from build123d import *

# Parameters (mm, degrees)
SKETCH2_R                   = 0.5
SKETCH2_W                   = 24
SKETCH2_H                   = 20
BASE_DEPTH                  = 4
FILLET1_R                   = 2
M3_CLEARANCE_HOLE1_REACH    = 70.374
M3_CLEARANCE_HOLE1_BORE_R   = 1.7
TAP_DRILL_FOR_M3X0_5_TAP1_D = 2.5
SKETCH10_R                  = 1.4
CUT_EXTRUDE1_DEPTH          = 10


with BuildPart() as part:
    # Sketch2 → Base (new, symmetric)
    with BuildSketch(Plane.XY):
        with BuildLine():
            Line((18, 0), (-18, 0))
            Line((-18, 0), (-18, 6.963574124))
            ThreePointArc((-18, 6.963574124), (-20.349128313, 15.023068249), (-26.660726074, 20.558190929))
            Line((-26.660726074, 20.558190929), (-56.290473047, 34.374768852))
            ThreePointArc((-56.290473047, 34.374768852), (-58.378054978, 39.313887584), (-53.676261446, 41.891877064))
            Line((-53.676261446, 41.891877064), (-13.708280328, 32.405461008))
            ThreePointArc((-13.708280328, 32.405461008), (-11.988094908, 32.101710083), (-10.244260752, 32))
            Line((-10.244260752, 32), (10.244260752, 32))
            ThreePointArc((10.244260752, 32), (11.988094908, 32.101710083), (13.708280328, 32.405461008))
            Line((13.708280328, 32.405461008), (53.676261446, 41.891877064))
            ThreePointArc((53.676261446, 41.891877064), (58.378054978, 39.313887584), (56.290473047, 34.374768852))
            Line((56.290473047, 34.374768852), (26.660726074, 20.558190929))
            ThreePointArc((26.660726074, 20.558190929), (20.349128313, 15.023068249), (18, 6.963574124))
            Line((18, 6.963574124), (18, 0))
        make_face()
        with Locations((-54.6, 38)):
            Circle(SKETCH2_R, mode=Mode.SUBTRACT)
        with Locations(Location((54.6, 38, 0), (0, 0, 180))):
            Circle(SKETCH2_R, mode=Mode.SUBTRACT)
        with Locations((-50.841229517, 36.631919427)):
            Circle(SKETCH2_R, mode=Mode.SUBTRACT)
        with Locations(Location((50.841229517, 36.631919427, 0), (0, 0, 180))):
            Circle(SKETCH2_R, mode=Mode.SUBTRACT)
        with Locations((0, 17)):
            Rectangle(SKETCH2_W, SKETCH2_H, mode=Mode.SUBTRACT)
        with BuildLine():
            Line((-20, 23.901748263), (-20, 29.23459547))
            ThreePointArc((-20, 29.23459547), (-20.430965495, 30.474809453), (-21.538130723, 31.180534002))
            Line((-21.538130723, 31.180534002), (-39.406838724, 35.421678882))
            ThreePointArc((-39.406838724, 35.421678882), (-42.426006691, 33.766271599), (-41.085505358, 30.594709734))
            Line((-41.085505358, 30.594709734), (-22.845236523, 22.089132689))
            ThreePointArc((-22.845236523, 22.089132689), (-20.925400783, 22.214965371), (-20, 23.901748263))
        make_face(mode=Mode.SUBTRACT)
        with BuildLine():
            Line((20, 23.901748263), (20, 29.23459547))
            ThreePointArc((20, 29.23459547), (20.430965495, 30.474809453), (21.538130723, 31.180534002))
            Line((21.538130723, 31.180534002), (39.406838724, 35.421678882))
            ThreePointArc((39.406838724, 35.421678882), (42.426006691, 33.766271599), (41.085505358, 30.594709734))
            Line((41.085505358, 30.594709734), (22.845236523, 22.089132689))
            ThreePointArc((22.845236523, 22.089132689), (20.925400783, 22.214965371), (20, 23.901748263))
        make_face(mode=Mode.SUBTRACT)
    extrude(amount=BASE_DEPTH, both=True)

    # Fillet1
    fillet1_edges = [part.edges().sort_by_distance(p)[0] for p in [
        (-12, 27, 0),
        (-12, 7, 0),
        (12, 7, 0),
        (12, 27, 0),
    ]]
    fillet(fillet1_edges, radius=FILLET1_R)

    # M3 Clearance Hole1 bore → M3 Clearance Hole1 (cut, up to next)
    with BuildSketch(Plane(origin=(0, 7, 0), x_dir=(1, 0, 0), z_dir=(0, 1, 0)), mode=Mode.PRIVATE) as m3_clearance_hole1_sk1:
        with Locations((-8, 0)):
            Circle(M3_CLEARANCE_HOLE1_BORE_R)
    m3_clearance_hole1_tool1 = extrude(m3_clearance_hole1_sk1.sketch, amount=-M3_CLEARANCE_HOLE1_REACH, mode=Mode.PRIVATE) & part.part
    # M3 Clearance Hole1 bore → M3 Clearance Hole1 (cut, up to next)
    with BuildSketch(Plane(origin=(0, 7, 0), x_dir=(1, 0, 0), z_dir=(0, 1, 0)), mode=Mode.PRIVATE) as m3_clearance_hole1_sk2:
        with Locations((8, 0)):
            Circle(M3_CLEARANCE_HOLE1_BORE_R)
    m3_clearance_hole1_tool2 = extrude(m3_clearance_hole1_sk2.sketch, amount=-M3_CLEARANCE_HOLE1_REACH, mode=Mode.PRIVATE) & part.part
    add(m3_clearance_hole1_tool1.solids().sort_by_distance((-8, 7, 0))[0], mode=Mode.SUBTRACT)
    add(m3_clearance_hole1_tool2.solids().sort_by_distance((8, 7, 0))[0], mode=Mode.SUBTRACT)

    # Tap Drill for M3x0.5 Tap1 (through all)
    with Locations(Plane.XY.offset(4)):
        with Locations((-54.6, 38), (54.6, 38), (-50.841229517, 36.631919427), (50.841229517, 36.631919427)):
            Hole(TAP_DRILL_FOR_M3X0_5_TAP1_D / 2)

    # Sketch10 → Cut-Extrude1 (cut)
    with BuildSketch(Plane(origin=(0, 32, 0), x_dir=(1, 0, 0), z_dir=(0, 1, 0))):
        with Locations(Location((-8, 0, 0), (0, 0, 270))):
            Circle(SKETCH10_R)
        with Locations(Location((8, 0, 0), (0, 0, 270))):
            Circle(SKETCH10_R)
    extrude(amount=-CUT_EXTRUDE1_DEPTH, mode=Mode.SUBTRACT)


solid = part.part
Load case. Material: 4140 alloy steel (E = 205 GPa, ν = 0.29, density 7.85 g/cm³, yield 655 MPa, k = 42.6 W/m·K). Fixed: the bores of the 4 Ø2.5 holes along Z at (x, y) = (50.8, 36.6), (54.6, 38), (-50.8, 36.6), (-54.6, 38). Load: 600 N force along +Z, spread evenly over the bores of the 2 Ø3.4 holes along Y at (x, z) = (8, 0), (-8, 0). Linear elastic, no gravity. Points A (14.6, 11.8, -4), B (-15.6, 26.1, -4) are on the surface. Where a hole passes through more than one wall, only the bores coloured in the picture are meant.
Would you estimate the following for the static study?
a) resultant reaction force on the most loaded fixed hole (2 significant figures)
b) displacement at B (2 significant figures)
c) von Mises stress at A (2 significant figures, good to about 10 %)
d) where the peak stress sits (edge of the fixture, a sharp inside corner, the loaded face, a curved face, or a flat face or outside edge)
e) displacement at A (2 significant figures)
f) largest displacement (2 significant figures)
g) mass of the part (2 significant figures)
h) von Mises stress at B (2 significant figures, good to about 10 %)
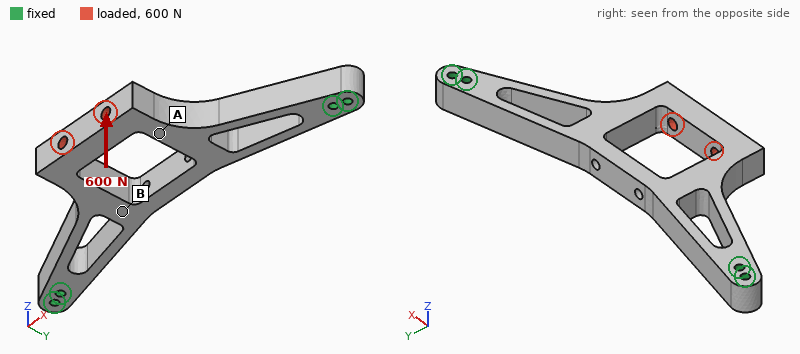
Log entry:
600 N
0.082 mm
41 MPa
a curved face
0.21 mm
0.33 mm
83 g
86 MPa
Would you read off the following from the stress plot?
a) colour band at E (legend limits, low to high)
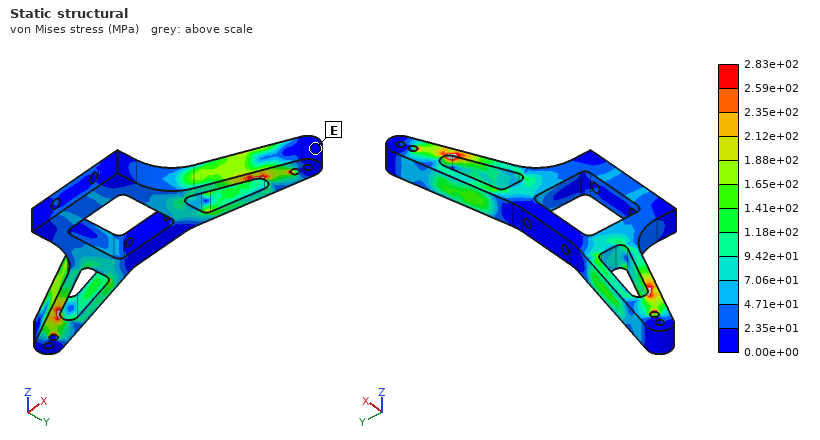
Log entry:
0.00e+00 to 2.35e+01 MPa
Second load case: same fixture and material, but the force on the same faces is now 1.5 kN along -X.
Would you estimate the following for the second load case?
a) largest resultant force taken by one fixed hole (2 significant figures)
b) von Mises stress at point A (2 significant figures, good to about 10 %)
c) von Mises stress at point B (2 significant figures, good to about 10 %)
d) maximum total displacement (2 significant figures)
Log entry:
700 N
36 MPa
11 MPa
21 µm
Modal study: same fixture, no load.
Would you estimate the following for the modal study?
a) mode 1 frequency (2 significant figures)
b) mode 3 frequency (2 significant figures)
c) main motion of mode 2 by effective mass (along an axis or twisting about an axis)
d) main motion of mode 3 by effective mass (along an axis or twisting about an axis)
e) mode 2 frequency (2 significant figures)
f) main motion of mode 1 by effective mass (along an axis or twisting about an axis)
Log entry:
1500 Hz
4900 Hz
along Z
along Y
4700 Hz
along Z
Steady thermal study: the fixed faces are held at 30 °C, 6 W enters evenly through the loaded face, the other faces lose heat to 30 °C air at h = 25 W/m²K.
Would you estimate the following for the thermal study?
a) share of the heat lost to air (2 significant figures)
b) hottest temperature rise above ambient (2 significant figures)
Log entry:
53 %
47 K
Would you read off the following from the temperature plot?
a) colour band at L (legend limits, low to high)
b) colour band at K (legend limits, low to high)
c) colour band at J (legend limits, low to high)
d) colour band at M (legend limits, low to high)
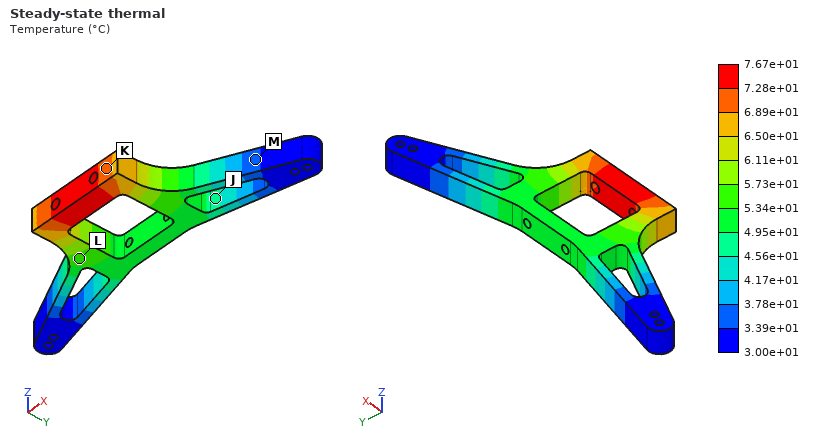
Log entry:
5.34e+01 to 5.73e+01 °C
6.89e+01 to 7.28e+01 °C
4.56e+01 to 4.95e+01 °C
3.39e+01 to 3.78e+01 °C
